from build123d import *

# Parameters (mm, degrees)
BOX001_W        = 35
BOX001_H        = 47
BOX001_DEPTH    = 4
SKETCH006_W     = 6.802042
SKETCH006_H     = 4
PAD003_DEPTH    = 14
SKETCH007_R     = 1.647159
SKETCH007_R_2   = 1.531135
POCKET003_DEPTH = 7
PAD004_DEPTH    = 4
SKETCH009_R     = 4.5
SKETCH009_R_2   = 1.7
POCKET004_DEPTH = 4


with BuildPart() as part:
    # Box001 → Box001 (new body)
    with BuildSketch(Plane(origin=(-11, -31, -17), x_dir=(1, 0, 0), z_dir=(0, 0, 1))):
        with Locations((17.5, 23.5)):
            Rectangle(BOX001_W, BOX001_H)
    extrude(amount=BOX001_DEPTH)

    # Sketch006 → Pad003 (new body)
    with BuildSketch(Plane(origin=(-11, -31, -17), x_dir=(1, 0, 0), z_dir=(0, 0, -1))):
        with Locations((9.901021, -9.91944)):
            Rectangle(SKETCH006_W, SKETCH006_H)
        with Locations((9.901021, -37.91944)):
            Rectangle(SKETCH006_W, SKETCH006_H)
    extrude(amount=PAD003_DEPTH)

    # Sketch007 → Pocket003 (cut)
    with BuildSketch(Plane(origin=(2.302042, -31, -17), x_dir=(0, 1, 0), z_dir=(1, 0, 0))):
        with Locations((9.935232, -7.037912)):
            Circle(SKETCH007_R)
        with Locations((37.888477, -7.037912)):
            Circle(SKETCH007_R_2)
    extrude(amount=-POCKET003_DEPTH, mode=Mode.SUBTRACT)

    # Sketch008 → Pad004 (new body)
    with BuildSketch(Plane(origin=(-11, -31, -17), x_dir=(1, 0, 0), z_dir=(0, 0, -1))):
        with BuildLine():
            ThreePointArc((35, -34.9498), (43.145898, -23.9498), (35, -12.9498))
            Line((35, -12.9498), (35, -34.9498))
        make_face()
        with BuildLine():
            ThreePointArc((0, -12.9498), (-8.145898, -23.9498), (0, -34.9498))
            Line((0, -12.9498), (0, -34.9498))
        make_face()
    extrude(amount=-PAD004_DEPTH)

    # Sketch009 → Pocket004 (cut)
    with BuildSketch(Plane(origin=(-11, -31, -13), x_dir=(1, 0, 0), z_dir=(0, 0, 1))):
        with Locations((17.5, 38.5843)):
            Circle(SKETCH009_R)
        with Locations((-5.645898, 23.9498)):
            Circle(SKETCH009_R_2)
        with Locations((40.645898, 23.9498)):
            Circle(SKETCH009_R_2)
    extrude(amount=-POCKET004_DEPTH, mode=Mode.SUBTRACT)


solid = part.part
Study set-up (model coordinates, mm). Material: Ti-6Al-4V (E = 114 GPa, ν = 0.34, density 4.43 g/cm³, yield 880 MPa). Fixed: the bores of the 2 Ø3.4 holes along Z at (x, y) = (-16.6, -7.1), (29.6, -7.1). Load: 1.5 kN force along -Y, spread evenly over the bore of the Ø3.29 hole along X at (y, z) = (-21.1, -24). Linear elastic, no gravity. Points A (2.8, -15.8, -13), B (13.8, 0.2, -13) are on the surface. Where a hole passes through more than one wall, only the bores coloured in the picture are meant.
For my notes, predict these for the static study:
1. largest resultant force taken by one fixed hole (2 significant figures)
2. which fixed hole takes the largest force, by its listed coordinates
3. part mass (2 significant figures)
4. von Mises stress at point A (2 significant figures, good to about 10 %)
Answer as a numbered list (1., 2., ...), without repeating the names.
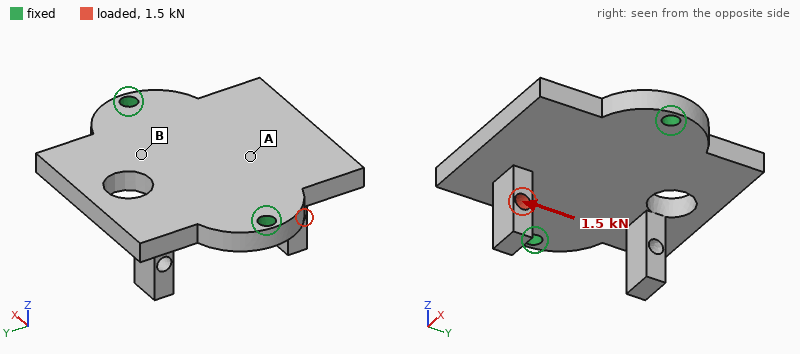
1. 1.0 kN
2. (-16.6, -7.1)
3. 35 g
4. 130 MPa
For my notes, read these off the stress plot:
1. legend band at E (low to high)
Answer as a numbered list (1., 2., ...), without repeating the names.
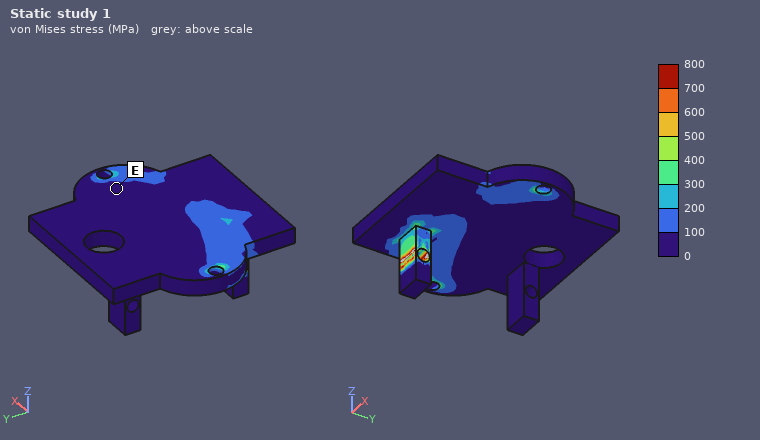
1. 0 to 100 MPa
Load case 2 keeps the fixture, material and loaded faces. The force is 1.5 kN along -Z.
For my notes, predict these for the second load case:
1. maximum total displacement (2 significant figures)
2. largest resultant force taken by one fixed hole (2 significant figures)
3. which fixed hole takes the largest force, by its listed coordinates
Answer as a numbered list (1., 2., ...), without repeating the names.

1. 0.31 mm
2. 1.1 kN
3. (-16.6, -7.1)
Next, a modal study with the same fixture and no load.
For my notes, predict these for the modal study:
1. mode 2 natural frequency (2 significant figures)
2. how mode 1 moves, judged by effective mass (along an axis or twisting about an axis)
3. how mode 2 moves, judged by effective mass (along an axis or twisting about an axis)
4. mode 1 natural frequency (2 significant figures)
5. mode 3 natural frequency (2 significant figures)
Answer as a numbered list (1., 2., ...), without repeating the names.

1. 4700 Hz
2. twisting about X
3. along Z
4. 3300 Hz
5. 8900 Hz
